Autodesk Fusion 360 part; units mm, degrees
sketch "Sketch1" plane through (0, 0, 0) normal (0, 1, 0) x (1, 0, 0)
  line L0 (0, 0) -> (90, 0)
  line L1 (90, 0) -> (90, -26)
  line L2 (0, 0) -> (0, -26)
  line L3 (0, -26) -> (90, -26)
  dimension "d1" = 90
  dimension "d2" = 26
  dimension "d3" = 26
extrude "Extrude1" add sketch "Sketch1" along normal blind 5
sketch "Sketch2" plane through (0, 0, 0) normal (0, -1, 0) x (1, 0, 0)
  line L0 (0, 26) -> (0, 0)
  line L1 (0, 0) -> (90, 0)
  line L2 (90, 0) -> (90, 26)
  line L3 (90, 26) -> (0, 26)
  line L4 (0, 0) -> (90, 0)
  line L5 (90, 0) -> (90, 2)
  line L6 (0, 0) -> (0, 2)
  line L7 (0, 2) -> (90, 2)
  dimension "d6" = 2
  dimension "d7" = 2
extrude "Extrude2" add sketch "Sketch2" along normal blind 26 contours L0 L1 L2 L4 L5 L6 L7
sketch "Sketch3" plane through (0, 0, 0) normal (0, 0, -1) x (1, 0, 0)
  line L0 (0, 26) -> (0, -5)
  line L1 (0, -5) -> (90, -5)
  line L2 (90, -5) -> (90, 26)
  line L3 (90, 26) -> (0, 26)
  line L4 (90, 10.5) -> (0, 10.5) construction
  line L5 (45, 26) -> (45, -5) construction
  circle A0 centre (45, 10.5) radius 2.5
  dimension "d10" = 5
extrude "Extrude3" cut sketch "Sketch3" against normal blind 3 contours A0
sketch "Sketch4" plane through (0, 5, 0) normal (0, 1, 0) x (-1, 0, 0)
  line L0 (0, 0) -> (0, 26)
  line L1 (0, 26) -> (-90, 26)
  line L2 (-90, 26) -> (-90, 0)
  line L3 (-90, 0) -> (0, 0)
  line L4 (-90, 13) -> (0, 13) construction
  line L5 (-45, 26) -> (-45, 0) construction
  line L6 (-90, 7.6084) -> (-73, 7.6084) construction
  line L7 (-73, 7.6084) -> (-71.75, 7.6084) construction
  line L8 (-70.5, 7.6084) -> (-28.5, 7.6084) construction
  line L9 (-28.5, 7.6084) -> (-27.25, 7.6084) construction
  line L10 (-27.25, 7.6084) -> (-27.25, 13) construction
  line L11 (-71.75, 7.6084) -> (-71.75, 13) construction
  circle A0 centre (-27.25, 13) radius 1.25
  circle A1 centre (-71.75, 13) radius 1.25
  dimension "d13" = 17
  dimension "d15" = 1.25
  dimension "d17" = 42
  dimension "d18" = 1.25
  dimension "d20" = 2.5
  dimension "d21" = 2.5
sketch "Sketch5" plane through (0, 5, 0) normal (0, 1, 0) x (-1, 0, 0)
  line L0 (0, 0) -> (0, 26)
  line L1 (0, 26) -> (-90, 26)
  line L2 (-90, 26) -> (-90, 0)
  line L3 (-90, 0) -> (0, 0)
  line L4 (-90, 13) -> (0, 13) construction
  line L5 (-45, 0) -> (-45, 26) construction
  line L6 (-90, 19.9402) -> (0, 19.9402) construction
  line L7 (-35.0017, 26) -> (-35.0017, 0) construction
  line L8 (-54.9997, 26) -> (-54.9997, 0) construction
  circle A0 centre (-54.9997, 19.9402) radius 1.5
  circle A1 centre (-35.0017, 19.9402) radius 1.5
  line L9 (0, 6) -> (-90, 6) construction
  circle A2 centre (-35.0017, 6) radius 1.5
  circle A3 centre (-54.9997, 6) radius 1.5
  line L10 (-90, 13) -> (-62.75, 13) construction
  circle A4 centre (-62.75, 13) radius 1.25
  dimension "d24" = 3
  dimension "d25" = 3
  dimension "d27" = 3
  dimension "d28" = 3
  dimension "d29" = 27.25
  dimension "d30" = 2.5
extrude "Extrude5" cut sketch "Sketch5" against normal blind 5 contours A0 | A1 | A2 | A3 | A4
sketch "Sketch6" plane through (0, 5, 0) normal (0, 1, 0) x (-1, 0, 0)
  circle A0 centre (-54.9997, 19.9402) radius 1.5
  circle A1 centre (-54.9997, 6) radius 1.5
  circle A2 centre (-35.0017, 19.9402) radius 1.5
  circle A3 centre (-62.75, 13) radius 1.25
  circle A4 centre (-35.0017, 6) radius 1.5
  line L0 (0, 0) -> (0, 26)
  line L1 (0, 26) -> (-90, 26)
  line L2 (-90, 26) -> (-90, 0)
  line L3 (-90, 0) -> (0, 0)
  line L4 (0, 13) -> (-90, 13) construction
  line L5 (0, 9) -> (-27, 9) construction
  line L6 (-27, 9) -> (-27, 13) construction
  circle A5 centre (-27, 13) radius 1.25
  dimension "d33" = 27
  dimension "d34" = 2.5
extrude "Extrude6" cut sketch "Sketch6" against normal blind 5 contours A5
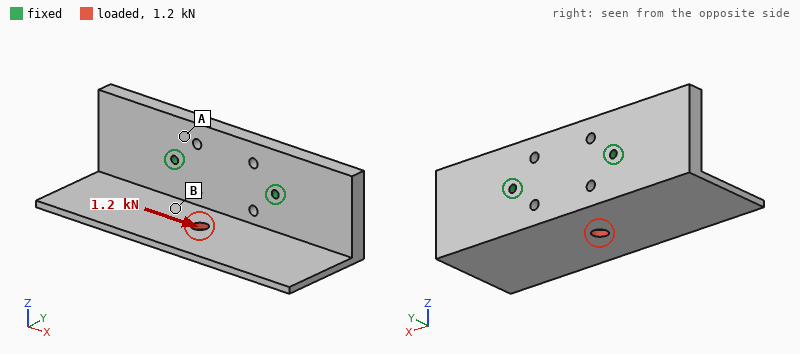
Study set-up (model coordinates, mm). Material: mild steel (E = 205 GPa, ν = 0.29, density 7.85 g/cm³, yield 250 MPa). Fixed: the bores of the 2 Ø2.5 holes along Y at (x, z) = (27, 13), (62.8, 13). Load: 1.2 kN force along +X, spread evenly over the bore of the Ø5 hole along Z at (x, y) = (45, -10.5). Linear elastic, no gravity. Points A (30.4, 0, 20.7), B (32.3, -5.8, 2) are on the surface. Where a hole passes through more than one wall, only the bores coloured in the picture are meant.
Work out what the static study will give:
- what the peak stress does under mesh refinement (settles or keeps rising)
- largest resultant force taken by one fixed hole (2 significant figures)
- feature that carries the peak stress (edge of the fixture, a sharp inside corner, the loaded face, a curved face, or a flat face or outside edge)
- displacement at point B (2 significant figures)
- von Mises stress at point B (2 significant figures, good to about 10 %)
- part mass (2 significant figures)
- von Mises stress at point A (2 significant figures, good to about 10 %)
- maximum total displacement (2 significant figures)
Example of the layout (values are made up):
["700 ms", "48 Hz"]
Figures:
["keeps rising", "800 N", "edge of the fixture", "6.1 µm", "24 MPa", "130 g", "9.7 MPa", "23 µm"]
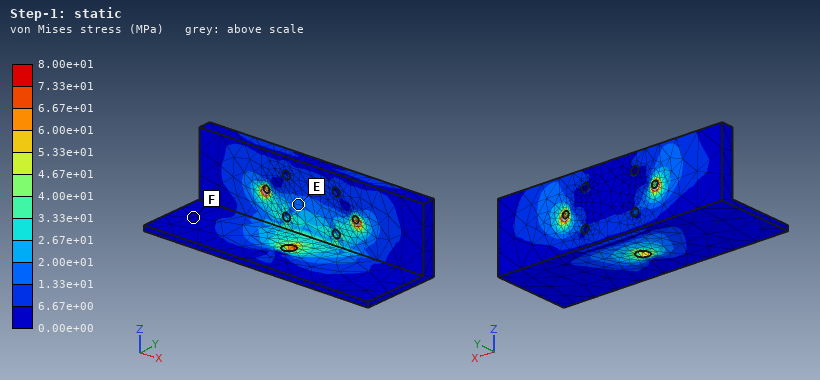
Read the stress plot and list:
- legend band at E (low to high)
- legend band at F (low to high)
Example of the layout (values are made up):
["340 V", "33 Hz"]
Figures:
["1.33e+01 to 2.00e+01 MPa", "0.00e+00 to 6.67e+00 MPa"]
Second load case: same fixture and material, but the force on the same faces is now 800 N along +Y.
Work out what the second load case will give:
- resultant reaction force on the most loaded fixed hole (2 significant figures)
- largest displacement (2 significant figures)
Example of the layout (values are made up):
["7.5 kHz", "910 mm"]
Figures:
["410 N", "25 µm"]
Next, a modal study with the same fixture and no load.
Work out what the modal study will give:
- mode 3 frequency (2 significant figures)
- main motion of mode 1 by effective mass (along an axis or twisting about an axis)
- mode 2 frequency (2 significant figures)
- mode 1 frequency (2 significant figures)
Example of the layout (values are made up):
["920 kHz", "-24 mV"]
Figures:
["4000 Hz", "along Z", "2600 Hz", "2100 Hz"]
